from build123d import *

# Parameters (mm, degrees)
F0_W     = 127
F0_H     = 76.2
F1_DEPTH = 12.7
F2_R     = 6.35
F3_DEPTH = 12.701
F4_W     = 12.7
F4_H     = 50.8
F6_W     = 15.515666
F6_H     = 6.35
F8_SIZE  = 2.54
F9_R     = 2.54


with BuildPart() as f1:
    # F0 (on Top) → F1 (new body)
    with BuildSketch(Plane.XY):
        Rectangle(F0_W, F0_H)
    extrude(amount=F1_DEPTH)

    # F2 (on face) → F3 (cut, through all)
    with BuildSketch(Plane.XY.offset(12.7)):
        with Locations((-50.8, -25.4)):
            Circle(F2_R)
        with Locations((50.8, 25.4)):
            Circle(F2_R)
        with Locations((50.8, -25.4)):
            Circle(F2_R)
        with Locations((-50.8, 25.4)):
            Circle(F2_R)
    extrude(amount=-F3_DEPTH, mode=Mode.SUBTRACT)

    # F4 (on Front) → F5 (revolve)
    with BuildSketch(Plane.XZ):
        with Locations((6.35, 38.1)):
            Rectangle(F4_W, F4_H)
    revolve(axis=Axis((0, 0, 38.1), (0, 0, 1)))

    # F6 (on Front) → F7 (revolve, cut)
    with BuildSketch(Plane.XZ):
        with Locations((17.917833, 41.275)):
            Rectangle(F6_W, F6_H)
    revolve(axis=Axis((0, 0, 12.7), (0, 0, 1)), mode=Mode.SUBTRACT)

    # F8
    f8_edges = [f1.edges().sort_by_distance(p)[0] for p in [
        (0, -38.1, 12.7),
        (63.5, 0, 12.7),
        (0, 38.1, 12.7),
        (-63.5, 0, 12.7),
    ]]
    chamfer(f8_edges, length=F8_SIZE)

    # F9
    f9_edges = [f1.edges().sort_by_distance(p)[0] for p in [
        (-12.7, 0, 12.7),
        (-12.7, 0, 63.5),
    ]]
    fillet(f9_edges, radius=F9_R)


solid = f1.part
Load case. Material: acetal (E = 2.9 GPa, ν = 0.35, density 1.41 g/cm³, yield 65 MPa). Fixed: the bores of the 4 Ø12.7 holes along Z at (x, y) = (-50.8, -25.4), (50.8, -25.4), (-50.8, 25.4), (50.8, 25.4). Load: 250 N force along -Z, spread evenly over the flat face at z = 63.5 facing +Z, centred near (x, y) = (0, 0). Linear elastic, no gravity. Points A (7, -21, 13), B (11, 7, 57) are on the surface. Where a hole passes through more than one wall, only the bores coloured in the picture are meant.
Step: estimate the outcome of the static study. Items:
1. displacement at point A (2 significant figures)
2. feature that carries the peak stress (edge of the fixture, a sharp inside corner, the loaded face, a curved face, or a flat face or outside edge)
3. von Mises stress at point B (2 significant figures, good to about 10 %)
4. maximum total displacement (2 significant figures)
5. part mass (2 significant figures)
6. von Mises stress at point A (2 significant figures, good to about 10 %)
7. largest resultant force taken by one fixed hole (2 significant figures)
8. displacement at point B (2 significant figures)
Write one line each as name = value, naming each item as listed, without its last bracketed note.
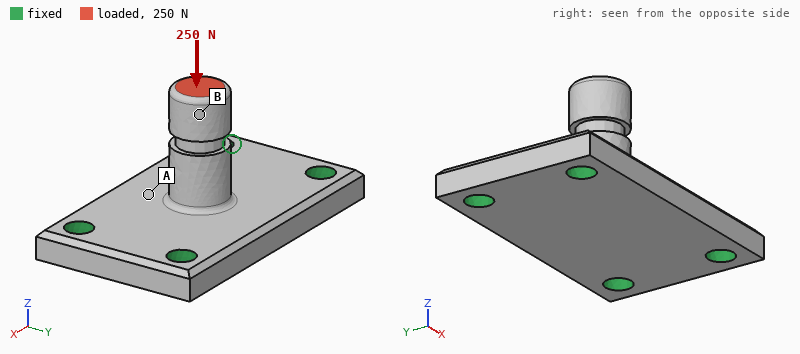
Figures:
displacement at point A = 29 µm
feature that carries the peak stress = a curved face
von Mises stress at point B = 0.33 MPa
maximum total displacement = 44 µm
part mass = 200 g
von Mises stress at point A = 0.76 MPa
largest resultant force taken by one fixed hole = 63 N
displacement at point B = 42 µm
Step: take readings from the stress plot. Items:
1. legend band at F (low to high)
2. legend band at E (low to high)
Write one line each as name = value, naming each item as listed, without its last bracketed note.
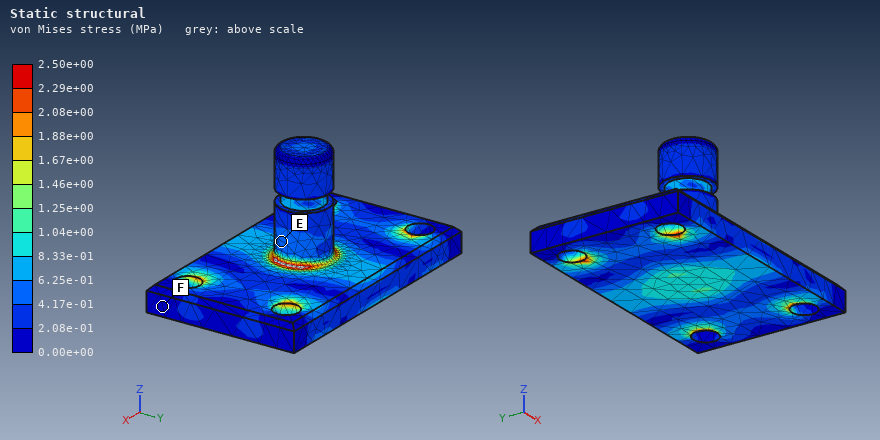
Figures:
legend band at F = 0.00e+00 to 2.08e-01 MPa
legend band at E = 4.17e-01 to 6.25e-01 MPa
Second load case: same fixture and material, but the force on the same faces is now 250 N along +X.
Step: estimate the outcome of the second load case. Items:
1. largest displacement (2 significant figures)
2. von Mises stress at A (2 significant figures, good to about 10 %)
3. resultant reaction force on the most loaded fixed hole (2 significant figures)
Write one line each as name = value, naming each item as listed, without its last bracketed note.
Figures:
largest displacement = 0.40 mm
von Mises stress at A = 1.3 MPa
resultant reaction force on the most loaded fixed hole = 120 N
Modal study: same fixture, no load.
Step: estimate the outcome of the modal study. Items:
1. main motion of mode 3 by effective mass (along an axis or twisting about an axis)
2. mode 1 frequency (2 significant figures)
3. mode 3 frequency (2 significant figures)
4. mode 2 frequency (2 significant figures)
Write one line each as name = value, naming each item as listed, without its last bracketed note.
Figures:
main motion of mode 3 by effective mass = along Z
mode 1 frequency = 1100 Hz
mode 3 frequency = 1500 Hz
mode 2 frequency = 1200 Hz
